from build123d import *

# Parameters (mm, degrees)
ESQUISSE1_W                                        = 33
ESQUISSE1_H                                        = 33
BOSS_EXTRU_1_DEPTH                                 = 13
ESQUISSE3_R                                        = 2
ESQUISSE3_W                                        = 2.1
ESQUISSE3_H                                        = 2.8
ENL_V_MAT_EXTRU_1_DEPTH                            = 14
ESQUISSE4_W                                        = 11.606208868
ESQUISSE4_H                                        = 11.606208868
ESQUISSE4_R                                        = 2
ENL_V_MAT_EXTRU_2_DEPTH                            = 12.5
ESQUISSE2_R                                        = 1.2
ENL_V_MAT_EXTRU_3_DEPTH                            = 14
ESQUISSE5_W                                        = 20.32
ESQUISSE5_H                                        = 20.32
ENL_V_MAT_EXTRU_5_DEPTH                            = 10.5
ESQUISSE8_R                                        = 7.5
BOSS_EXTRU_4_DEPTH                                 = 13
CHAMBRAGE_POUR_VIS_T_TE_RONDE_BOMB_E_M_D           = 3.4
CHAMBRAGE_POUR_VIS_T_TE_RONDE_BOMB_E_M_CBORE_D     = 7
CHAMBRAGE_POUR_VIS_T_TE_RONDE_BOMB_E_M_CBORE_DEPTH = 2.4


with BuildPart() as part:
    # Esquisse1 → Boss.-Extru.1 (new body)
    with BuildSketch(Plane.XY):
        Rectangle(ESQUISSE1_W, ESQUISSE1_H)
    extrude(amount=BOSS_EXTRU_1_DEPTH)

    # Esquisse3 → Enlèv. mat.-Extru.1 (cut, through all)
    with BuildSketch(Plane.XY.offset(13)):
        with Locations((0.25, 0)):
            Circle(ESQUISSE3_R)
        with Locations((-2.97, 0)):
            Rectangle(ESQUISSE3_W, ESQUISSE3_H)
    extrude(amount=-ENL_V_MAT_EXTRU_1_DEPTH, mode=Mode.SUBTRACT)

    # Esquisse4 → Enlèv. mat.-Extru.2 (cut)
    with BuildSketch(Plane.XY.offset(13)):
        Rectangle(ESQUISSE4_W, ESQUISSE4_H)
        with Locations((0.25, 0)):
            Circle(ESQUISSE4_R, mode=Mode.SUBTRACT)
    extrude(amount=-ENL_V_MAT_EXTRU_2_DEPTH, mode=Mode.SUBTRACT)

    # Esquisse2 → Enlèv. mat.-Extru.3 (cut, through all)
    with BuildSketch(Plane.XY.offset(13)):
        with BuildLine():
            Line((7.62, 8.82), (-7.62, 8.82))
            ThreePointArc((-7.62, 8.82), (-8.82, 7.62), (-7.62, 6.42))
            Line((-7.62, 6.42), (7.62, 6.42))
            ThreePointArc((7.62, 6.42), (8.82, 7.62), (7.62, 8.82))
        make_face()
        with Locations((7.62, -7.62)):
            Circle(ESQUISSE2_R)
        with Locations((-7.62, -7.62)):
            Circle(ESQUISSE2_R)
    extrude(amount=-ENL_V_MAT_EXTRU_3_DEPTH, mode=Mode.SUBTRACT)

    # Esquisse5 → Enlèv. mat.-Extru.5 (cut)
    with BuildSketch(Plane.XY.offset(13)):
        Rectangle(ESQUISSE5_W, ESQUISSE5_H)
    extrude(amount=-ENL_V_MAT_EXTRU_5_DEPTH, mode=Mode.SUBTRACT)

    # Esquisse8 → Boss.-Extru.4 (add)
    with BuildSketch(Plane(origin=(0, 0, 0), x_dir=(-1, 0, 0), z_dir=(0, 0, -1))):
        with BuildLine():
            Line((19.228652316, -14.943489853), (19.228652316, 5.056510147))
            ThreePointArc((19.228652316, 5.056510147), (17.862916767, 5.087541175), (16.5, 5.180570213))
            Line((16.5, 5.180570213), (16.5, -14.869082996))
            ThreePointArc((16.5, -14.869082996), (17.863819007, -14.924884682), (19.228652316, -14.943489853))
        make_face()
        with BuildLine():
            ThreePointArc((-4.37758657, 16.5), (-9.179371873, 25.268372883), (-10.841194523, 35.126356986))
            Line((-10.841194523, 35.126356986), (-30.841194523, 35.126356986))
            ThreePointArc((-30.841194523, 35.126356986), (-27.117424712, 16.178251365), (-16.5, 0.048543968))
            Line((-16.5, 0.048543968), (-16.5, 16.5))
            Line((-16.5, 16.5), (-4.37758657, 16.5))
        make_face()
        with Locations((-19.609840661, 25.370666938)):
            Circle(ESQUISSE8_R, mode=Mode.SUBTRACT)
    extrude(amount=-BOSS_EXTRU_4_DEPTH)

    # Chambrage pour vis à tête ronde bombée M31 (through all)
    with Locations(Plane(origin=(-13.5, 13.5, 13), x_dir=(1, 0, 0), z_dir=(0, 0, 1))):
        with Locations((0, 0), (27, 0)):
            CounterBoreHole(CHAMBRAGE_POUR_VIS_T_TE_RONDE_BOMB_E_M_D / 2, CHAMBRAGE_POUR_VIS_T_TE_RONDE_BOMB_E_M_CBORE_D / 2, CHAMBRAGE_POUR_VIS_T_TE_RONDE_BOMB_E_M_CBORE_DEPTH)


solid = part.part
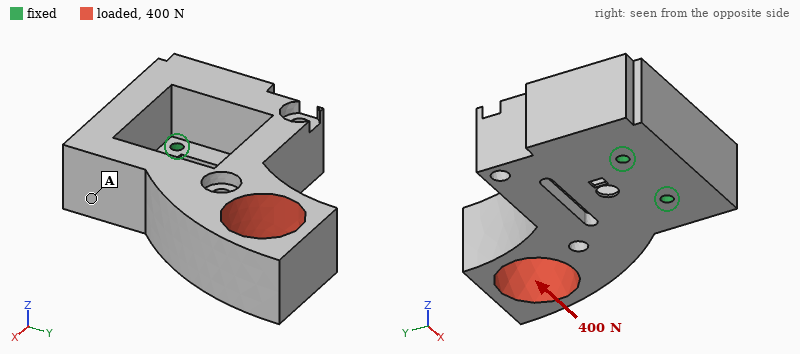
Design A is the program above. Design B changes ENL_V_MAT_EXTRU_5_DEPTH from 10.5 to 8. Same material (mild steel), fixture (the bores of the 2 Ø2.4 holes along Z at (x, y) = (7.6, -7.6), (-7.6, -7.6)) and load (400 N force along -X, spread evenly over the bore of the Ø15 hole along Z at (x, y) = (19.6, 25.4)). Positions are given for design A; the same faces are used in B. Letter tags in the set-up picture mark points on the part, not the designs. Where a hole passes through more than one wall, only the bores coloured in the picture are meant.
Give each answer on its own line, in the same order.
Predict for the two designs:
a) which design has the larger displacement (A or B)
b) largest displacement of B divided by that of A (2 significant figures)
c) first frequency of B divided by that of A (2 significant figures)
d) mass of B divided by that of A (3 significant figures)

A
0.73
1.8
1.04
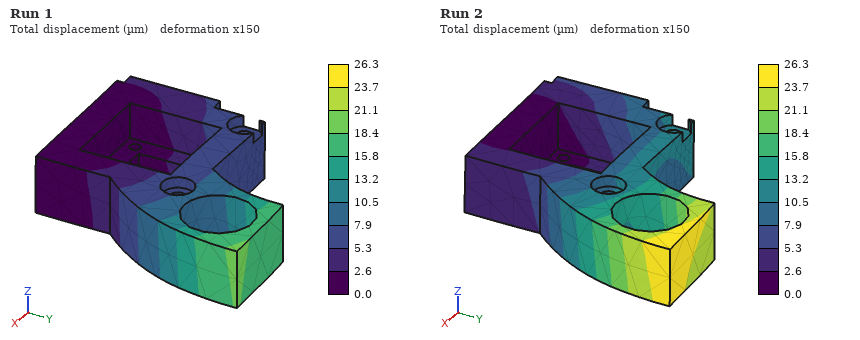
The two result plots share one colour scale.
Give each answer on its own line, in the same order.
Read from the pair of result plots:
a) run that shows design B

Run 1
